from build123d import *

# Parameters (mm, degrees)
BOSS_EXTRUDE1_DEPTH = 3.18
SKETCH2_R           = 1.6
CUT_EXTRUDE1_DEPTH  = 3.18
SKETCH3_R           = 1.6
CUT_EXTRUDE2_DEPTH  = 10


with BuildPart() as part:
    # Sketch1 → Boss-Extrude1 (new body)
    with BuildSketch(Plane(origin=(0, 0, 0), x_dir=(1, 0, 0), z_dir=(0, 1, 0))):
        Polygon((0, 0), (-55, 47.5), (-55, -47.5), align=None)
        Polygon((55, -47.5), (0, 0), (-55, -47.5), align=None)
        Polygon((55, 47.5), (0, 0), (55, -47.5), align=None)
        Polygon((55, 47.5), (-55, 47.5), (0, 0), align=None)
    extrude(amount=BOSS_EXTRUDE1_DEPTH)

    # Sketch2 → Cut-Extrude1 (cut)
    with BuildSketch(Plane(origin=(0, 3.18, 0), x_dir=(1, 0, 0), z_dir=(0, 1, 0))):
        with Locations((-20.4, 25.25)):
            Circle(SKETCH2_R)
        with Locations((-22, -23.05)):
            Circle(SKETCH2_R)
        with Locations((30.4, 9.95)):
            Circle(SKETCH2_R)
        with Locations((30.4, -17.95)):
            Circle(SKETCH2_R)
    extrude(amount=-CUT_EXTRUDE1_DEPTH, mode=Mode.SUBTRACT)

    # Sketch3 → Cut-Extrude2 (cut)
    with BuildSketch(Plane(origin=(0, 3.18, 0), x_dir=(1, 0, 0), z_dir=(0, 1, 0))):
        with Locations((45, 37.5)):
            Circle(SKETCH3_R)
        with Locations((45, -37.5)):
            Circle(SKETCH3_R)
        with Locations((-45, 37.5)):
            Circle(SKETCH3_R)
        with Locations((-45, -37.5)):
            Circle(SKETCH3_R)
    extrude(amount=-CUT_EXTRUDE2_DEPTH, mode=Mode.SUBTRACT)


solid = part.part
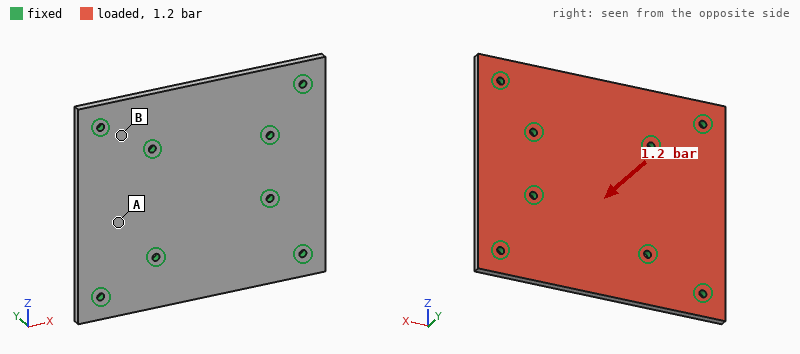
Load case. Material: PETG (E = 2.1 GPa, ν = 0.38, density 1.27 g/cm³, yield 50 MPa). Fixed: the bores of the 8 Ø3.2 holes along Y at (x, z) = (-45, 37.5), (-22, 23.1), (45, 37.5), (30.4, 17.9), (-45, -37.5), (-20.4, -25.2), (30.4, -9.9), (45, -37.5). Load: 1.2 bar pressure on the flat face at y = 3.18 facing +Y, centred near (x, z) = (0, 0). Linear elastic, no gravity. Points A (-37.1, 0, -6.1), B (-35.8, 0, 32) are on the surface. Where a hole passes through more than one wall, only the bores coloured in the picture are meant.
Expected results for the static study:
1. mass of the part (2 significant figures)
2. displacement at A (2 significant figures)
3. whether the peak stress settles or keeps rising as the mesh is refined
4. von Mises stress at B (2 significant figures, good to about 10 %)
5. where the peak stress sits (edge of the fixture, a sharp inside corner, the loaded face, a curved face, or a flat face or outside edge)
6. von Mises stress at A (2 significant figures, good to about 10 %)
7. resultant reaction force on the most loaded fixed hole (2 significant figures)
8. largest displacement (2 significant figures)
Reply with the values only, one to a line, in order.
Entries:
42 g
0.67 mm
keeps rising
12 MPa
edge of the fixture
7.6 MPa
250 N
1.4 mm
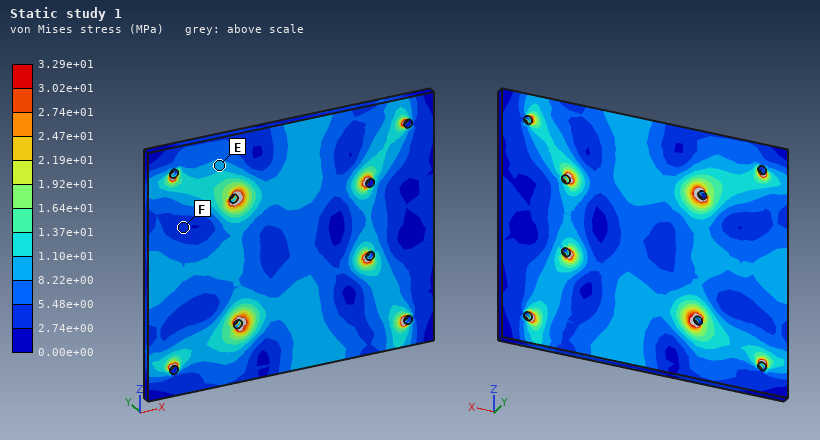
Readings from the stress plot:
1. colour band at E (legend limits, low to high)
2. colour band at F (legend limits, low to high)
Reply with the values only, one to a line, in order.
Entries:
8.22e+00 to 1.10e+01 MPa
2.74e+00 to 5.48e+00 MPa
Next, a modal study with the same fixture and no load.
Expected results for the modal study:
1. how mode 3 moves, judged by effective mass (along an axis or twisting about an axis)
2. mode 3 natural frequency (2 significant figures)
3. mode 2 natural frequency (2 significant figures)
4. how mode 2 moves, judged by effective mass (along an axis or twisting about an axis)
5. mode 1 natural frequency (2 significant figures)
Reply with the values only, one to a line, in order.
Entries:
along Y
1000 Hz
940 Hz
twisting about X
890 Hz
